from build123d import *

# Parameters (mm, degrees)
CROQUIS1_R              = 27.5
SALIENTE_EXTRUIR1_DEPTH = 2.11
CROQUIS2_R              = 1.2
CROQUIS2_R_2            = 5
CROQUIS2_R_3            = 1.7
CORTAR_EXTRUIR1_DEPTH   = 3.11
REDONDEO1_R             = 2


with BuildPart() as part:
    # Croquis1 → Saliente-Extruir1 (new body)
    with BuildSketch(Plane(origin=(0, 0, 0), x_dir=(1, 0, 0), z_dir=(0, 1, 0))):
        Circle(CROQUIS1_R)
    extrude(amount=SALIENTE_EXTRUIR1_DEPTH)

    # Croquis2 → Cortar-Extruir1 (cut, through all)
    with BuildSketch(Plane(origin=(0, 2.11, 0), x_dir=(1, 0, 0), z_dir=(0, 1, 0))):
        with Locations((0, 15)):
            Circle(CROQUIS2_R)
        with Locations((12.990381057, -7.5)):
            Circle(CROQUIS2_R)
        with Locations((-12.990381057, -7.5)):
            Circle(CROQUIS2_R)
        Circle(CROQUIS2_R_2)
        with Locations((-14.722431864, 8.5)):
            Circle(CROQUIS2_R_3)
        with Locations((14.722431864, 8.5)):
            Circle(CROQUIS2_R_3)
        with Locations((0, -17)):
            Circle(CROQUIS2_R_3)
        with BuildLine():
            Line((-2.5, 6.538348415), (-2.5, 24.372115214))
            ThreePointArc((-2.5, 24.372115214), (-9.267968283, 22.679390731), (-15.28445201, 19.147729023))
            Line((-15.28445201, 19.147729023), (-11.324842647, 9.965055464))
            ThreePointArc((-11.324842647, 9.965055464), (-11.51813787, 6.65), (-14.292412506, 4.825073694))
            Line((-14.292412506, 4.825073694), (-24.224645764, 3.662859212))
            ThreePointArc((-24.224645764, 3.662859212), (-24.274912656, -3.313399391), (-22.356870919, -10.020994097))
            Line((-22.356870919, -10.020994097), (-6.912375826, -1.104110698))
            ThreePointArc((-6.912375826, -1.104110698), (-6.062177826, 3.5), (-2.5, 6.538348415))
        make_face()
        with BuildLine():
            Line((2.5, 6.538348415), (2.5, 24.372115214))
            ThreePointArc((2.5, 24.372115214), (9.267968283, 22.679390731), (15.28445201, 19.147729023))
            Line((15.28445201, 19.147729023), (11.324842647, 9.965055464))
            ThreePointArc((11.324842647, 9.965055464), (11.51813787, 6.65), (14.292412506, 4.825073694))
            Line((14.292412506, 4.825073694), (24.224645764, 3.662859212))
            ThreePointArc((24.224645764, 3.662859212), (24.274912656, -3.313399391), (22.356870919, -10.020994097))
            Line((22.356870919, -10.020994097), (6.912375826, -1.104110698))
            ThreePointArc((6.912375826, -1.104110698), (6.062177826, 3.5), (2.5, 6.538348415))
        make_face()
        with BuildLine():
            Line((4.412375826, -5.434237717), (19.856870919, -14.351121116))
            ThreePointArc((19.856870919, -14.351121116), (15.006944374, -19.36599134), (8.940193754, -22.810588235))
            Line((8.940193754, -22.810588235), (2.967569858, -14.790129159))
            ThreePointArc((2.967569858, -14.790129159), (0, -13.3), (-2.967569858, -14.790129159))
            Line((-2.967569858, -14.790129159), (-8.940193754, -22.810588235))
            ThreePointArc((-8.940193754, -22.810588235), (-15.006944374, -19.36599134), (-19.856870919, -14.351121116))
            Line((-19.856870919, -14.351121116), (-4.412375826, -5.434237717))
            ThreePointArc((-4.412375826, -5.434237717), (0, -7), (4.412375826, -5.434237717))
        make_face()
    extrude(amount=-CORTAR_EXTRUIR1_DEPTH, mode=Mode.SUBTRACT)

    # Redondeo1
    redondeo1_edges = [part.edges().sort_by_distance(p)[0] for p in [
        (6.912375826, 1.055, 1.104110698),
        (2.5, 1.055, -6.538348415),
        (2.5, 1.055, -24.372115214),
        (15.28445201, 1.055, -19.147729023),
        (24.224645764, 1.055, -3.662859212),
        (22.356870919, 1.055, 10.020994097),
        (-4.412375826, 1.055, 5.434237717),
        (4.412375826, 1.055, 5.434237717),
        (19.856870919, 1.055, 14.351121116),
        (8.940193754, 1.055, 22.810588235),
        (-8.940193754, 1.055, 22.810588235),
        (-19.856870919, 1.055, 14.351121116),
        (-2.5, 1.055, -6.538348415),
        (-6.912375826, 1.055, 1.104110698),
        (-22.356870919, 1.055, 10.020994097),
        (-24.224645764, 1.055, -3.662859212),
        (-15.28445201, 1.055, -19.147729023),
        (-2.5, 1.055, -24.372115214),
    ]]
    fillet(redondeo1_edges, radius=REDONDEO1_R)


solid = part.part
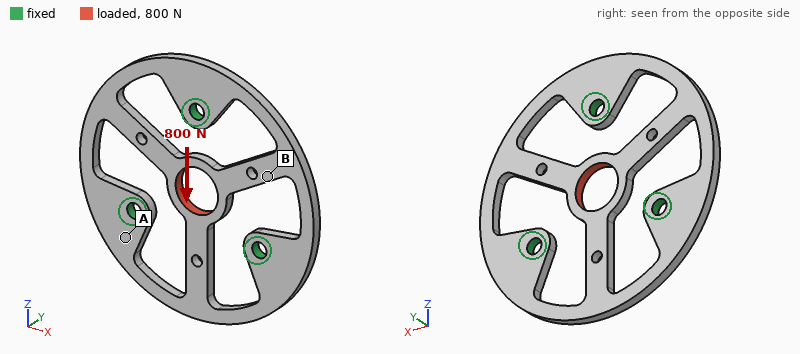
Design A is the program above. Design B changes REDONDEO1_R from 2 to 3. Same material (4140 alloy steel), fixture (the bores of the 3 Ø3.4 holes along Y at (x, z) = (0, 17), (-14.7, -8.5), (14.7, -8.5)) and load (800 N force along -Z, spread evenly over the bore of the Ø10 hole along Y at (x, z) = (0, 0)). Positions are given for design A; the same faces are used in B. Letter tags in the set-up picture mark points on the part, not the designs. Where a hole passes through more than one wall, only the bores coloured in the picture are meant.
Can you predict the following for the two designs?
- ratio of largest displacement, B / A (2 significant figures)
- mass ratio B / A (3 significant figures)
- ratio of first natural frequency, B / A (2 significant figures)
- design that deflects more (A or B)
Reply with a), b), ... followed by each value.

a) 0.89
b) 1.01
c) 1.0
d) A
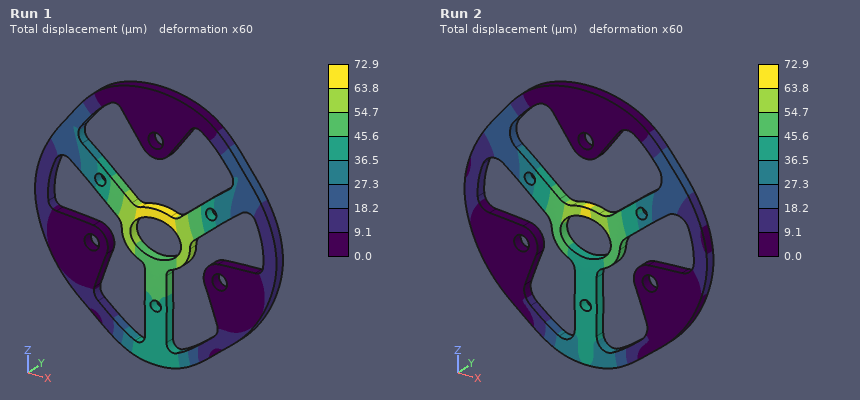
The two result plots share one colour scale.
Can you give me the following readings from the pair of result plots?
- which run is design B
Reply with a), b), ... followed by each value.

a) Run 2
